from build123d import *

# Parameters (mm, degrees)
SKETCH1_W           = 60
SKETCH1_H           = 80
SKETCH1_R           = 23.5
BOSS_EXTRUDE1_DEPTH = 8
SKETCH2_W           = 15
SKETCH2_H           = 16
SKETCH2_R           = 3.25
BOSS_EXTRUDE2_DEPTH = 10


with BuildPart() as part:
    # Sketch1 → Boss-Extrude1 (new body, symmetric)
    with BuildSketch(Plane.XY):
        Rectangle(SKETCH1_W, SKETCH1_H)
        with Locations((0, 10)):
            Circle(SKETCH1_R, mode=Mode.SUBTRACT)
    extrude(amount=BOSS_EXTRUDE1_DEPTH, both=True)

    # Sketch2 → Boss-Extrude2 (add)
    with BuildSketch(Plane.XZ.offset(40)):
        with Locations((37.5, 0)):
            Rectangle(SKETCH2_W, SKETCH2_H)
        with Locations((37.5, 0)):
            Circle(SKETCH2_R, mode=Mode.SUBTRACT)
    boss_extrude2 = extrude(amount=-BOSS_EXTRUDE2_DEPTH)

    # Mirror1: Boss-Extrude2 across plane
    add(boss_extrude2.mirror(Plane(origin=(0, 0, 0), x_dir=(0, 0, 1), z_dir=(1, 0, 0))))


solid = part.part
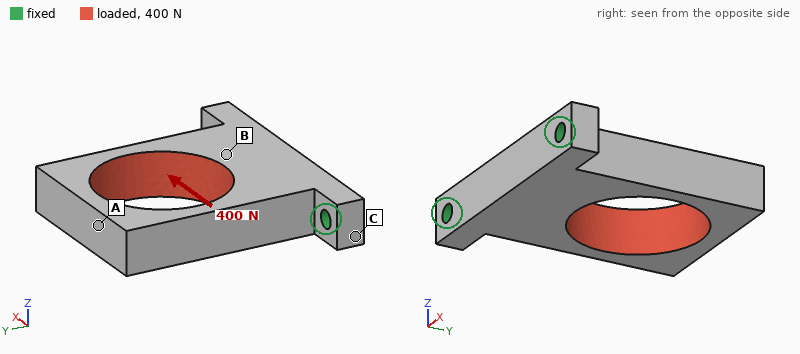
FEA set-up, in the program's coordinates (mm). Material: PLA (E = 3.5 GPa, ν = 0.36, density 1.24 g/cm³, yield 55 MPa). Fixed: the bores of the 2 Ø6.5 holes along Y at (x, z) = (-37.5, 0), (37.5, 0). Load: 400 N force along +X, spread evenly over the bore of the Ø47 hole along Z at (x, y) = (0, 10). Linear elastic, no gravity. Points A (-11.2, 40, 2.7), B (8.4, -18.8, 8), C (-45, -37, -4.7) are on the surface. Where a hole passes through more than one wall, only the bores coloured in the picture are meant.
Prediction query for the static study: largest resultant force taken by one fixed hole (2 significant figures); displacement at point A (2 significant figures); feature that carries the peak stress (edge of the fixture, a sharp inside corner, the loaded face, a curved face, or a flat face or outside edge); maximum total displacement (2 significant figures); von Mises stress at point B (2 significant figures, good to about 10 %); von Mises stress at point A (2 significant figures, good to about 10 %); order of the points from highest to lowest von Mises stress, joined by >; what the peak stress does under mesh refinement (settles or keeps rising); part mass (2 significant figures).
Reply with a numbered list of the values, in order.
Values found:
1. 340 N
2. 0.28 mm
3. edge of the fixture
4. 0.29 mm
5. 1.9 MPa
6. 3.0 MPa
7. A > B > C
8. keeps rising
9. 66 g
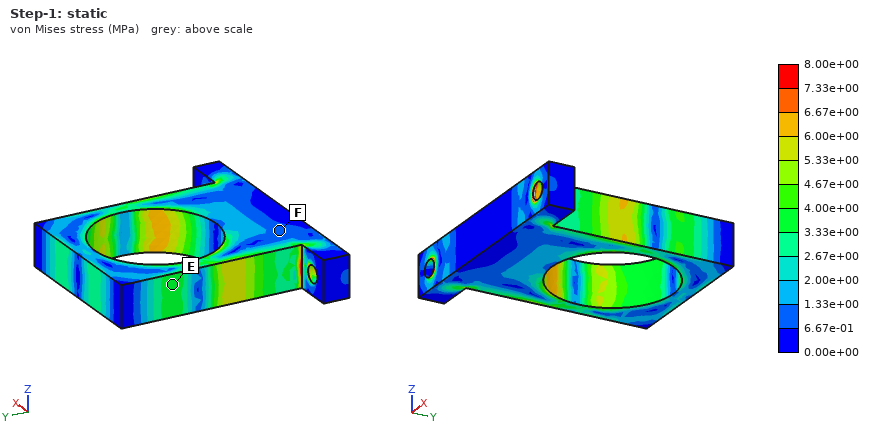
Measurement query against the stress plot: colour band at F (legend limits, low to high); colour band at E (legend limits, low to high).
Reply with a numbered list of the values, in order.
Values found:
1. 6.67e-01 to 1.33e+00 MPa
2. 3.33e+00 to 4.00e+00 MPa
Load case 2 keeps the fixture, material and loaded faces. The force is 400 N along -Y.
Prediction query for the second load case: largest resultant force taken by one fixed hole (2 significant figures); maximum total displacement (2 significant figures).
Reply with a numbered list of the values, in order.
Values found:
1. 210 N
2. 65 µm
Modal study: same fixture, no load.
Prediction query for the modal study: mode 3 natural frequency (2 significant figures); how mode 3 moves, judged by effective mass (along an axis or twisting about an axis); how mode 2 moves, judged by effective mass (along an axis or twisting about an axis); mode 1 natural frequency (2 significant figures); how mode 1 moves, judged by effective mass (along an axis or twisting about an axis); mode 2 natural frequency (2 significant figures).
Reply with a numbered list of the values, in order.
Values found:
1. 1200 Hz
2. twisting about Y
3. along X
4. 420 Hz
5. along Z
6. 1100 Hz
